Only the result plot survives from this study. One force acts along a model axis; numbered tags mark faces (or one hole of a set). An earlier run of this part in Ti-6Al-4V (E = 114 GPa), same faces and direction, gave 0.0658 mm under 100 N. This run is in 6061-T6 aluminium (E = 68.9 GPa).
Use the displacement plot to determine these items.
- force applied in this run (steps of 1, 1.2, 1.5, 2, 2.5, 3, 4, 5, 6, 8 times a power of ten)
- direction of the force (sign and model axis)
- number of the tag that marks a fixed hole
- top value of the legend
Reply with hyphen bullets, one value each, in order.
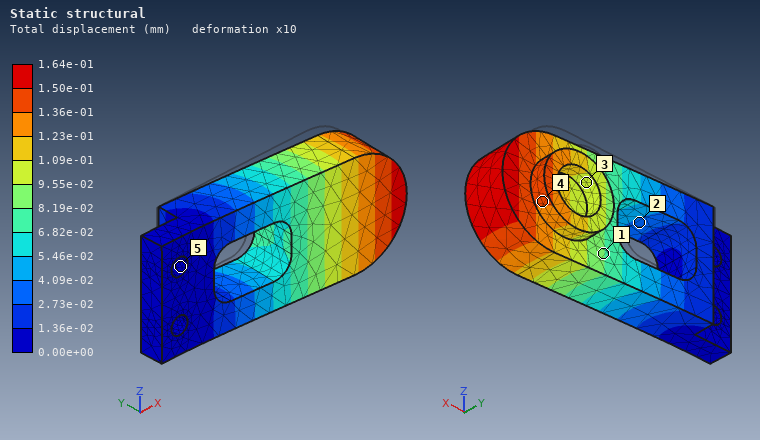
- 150 N
- -Y
- 5
- 1.64e-01 mm
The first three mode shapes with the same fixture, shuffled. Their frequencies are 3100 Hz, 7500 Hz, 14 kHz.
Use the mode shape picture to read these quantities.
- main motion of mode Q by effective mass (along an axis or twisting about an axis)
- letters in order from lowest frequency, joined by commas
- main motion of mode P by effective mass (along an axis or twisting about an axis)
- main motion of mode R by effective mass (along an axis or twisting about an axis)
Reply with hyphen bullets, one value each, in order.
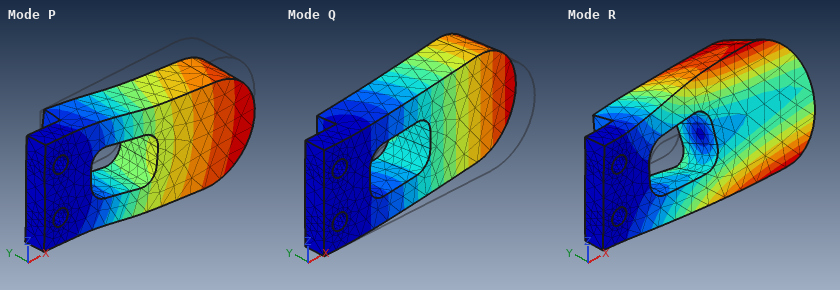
- along Y
- Q, P, R
- along Z
- twisting about X
